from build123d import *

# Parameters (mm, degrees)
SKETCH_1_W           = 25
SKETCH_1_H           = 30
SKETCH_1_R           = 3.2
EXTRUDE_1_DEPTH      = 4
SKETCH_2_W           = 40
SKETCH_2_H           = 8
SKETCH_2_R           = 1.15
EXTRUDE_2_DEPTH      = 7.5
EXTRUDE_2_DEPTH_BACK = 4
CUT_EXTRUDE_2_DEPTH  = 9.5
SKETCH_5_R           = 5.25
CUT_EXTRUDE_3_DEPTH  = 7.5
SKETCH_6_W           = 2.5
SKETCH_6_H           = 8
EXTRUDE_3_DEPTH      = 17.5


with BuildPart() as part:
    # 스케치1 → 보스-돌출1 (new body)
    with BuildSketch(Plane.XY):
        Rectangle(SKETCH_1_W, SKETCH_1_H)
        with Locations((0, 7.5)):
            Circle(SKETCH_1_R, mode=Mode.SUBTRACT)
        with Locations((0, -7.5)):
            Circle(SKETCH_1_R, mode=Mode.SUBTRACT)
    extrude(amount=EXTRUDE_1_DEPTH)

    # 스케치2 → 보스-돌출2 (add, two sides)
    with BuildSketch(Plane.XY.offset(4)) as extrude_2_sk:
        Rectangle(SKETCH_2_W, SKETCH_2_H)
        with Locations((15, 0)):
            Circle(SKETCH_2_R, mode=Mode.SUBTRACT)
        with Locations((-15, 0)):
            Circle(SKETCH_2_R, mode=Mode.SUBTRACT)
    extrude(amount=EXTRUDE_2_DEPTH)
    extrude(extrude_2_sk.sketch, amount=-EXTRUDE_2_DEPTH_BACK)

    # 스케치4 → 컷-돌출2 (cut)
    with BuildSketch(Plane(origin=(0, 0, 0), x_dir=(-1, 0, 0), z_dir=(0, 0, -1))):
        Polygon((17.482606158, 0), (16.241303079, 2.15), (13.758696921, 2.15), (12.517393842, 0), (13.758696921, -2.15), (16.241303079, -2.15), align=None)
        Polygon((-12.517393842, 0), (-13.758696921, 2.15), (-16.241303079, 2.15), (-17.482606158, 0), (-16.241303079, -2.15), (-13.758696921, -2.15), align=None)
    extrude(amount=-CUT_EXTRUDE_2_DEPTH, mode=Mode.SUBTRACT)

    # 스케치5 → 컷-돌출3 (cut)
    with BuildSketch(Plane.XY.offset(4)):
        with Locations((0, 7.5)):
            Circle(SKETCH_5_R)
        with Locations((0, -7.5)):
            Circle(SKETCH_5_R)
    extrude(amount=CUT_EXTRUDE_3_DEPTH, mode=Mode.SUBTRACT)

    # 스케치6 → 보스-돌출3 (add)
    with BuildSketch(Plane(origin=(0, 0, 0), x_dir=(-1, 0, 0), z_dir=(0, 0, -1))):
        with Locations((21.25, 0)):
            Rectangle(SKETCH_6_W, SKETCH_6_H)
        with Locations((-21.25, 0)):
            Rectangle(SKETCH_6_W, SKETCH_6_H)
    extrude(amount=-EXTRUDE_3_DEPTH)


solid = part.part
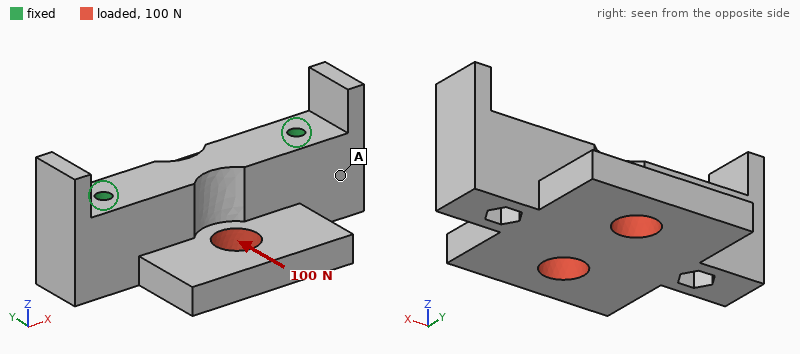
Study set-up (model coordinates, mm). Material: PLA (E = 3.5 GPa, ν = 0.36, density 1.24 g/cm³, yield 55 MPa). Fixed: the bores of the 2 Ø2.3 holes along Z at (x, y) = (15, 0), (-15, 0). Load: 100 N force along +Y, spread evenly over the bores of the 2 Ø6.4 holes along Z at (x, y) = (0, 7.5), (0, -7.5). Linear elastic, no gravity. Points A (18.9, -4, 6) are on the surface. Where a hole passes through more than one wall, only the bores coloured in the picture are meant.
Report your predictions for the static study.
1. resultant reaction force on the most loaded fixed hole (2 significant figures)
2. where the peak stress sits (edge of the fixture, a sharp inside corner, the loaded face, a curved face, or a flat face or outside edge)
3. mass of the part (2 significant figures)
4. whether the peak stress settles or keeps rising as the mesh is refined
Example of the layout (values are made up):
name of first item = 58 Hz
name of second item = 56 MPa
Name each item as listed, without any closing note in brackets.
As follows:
resultant reaction force on the most loaded fixed hole = 50 N
where the peak stress sits = edge of the fixture
mass of the part = 7.3 g
whether the peak stress settles or keeps rising as the mesh is refined = keeps rising
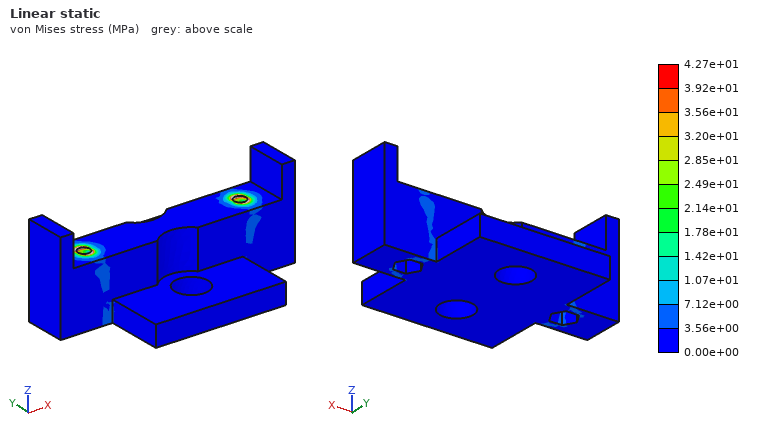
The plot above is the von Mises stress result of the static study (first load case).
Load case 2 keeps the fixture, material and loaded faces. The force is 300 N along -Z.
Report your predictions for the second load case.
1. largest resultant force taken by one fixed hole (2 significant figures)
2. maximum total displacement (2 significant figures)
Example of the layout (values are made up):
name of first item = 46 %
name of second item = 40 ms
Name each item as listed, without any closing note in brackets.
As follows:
largest resultant force taken by one fixed hole = 200 N
maximum total displacement = 0.14 mm
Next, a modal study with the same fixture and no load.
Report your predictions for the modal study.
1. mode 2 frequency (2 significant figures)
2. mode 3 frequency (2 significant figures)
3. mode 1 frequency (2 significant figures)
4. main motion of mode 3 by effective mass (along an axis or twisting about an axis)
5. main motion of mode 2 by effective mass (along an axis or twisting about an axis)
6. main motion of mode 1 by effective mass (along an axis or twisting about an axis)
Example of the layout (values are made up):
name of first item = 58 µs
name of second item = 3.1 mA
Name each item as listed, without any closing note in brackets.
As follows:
mode 2 frequency = 4400 Hz
mode 3 frequency = 4800 Hz
mode 1 frequency = 1500 Hz
main motion of mode 3 by effective mass = along Z
main motion of mode 2 by effective mass = twisting about Z
main motion of mode 1 by effective mass = along Y
